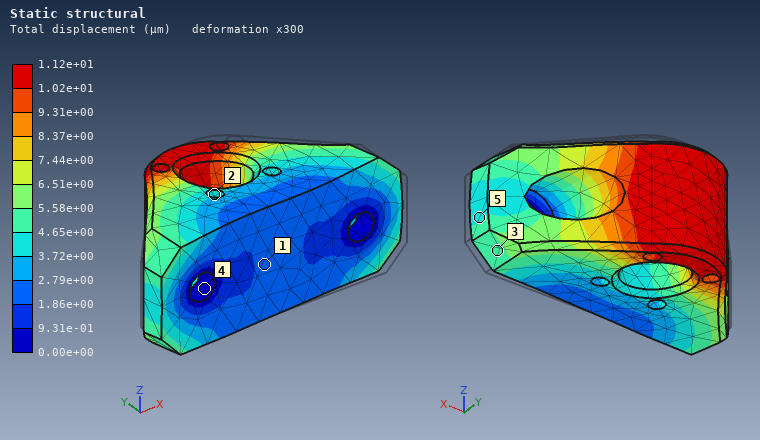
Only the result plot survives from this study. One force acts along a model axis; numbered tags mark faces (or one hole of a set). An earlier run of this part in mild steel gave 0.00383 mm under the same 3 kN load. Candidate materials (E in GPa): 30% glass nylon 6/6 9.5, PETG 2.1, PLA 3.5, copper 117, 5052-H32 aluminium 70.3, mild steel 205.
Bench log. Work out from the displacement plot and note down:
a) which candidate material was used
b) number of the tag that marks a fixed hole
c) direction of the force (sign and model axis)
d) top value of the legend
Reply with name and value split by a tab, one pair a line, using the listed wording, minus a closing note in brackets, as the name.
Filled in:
which candidate material was used	5052-H32 aluminium
number of the tag that marks a fixed hole	4
direction of the force	-X
top value of the legend	1.12e+01 µm
